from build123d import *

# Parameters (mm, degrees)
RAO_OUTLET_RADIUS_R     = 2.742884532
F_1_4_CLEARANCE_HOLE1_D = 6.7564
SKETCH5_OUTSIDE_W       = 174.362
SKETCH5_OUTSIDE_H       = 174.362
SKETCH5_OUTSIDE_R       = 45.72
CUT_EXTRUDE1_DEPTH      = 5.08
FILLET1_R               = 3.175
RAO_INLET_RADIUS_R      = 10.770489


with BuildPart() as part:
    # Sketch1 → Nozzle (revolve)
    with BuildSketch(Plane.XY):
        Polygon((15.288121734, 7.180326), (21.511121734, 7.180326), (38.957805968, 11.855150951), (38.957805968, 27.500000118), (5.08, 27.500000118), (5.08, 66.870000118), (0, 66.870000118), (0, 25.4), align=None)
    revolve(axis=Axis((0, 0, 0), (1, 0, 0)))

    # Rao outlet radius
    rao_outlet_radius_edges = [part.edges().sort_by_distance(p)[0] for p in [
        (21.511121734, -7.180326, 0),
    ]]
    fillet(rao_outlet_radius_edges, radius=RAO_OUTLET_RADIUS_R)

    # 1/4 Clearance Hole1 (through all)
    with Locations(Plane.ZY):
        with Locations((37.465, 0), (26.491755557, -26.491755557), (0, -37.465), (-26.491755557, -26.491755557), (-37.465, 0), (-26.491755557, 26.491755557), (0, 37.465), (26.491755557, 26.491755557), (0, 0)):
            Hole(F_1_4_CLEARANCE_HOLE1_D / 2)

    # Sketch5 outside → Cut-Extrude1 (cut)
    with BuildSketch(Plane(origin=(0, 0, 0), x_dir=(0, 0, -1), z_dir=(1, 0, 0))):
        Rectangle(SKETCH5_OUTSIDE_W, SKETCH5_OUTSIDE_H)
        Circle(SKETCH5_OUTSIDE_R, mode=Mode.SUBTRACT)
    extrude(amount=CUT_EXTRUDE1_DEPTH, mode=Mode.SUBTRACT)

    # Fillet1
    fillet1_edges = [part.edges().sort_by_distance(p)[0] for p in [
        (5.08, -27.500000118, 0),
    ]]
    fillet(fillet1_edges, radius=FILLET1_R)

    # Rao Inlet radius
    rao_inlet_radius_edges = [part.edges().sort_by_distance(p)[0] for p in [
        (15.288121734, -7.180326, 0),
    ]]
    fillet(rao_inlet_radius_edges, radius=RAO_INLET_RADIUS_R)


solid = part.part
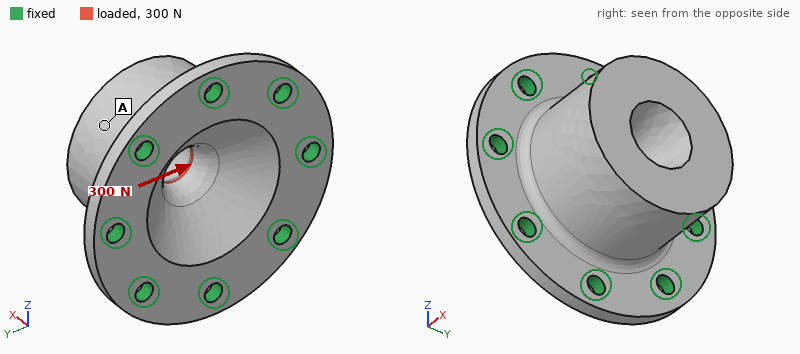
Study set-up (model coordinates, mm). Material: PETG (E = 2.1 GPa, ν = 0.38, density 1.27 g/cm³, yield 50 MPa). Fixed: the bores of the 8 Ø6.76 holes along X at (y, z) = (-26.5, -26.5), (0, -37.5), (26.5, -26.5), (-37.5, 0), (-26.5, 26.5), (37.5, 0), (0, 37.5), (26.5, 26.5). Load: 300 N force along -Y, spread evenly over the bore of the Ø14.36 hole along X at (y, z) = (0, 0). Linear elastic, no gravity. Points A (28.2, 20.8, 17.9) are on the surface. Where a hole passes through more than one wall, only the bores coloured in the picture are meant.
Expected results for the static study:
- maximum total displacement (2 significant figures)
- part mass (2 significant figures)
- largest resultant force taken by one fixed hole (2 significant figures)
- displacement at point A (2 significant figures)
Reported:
22 µm
120 g
73 N
17 µm
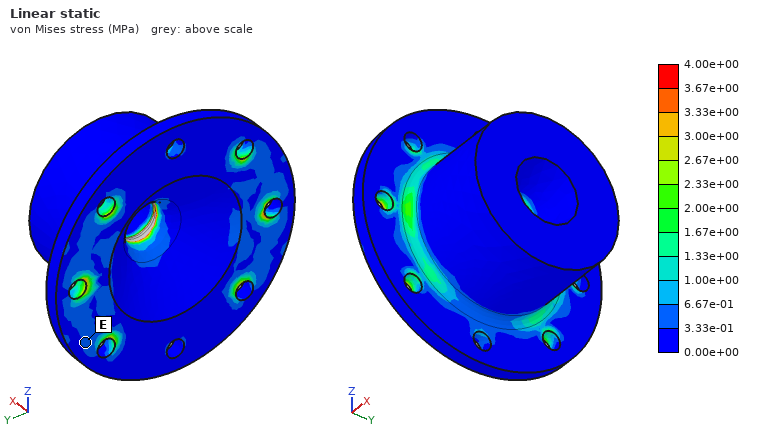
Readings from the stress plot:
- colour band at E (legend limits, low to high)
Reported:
3.33e-01 to 6.67e-01 MPa
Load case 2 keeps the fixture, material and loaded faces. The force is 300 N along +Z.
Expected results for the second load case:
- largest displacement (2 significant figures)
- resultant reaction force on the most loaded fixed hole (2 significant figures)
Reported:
22 µm
73 N
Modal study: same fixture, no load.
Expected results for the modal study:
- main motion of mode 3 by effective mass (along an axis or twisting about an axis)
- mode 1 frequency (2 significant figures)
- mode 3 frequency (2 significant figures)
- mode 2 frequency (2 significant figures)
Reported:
along X
2100 Hz
2400 Hz
2100 Hz
